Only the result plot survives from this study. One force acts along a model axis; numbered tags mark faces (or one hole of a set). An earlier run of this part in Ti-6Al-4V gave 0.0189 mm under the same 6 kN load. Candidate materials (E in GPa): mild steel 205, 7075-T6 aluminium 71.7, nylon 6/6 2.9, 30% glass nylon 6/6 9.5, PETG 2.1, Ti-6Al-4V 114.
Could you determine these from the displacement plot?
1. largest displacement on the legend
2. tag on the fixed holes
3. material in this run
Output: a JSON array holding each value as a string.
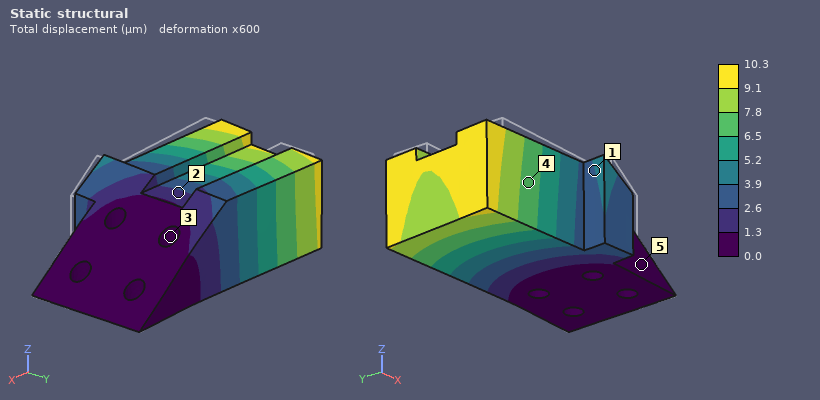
["10.3 µm", "3", "mild steel"]
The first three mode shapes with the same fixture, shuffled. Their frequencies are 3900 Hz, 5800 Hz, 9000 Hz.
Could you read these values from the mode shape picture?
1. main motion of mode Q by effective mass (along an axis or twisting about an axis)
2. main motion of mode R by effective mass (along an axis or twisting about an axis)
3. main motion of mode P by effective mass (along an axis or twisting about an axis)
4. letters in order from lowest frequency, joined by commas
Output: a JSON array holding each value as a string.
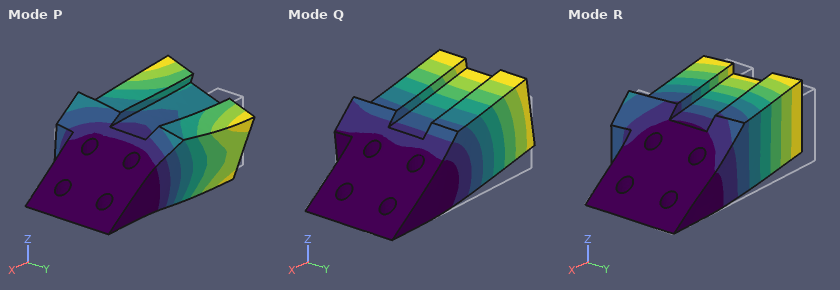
["along Z", "along Y", "twisting about X", "Q, R, P"]
